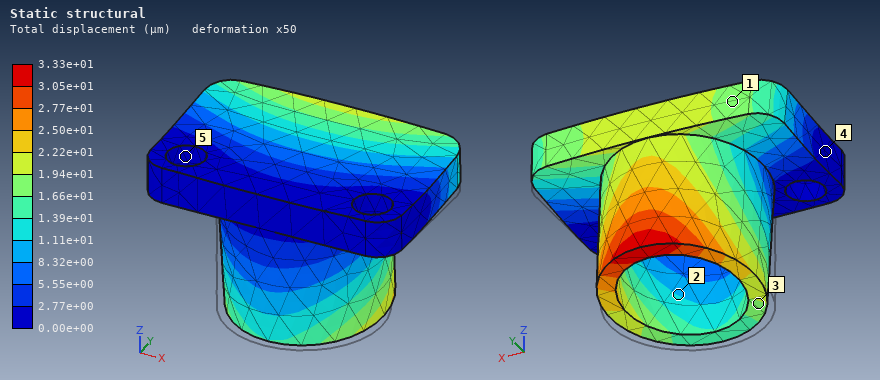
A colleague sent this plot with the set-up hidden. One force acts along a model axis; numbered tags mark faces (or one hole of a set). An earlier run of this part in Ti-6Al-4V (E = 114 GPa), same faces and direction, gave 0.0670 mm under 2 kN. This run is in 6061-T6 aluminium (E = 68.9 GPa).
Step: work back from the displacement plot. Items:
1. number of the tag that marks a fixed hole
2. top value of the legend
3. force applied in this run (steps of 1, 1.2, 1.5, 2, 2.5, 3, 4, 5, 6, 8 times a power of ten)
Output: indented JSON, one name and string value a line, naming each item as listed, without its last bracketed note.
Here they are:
{
  "number of the tag that marks a fixed hole": "5",
  "top value of the legend": "3.33e+01 µm",
  "force applied in this run": "600 N"
}
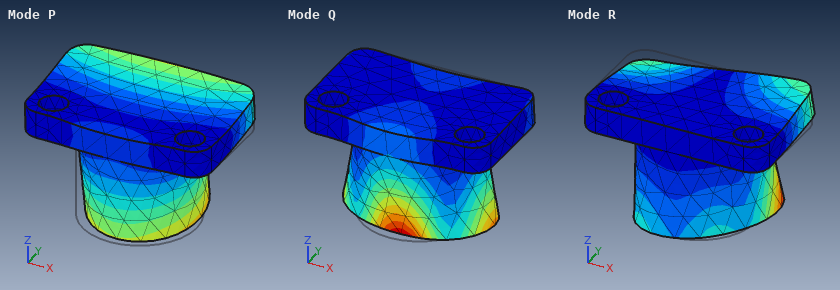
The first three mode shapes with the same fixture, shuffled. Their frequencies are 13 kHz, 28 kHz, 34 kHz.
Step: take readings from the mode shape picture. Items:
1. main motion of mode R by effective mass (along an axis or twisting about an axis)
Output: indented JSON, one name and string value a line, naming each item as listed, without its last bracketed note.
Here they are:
{
  "main motion of mode R by effective mass": "along X"
}
